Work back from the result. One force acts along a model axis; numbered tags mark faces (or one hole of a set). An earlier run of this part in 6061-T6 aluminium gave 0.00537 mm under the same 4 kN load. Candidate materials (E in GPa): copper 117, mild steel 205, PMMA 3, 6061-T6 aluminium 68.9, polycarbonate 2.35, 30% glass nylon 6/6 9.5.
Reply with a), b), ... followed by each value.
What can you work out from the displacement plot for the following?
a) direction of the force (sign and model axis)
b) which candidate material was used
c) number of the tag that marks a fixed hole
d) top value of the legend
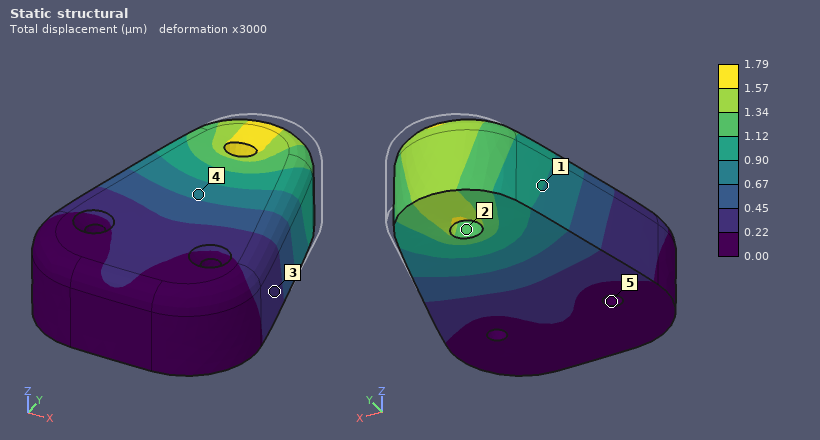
a) -Y
b) mild steel
c) 5
d) 1.79 µm
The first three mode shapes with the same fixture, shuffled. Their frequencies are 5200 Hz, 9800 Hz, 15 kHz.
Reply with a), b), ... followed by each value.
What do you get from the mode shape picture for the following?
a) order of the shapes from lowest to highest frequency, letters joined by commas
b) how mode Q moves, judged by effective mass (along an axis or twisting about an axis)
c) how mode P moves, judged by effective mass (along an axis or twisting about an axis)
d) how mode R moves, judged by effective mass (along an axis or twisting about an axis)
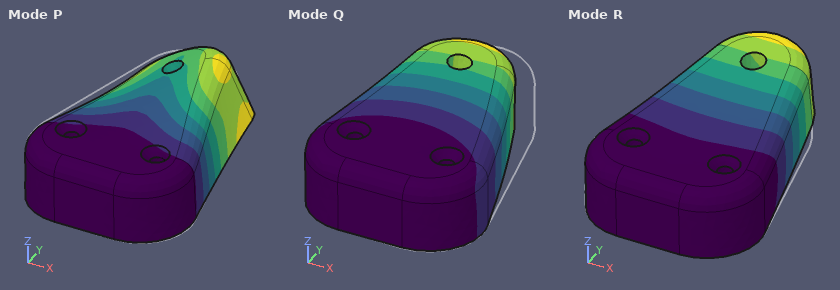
a) R, Q, P
b) along X
c) twisting about Y
d) along Z
